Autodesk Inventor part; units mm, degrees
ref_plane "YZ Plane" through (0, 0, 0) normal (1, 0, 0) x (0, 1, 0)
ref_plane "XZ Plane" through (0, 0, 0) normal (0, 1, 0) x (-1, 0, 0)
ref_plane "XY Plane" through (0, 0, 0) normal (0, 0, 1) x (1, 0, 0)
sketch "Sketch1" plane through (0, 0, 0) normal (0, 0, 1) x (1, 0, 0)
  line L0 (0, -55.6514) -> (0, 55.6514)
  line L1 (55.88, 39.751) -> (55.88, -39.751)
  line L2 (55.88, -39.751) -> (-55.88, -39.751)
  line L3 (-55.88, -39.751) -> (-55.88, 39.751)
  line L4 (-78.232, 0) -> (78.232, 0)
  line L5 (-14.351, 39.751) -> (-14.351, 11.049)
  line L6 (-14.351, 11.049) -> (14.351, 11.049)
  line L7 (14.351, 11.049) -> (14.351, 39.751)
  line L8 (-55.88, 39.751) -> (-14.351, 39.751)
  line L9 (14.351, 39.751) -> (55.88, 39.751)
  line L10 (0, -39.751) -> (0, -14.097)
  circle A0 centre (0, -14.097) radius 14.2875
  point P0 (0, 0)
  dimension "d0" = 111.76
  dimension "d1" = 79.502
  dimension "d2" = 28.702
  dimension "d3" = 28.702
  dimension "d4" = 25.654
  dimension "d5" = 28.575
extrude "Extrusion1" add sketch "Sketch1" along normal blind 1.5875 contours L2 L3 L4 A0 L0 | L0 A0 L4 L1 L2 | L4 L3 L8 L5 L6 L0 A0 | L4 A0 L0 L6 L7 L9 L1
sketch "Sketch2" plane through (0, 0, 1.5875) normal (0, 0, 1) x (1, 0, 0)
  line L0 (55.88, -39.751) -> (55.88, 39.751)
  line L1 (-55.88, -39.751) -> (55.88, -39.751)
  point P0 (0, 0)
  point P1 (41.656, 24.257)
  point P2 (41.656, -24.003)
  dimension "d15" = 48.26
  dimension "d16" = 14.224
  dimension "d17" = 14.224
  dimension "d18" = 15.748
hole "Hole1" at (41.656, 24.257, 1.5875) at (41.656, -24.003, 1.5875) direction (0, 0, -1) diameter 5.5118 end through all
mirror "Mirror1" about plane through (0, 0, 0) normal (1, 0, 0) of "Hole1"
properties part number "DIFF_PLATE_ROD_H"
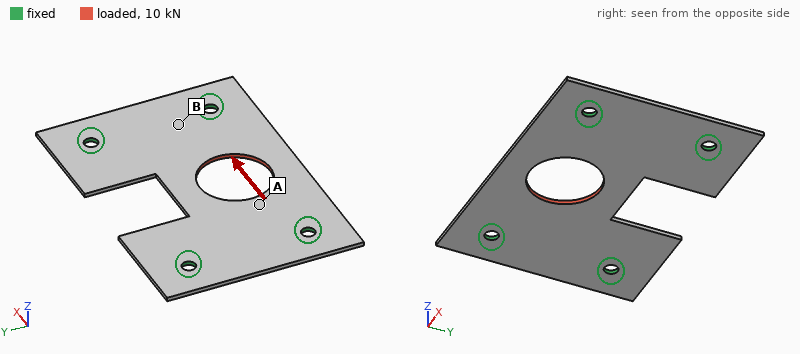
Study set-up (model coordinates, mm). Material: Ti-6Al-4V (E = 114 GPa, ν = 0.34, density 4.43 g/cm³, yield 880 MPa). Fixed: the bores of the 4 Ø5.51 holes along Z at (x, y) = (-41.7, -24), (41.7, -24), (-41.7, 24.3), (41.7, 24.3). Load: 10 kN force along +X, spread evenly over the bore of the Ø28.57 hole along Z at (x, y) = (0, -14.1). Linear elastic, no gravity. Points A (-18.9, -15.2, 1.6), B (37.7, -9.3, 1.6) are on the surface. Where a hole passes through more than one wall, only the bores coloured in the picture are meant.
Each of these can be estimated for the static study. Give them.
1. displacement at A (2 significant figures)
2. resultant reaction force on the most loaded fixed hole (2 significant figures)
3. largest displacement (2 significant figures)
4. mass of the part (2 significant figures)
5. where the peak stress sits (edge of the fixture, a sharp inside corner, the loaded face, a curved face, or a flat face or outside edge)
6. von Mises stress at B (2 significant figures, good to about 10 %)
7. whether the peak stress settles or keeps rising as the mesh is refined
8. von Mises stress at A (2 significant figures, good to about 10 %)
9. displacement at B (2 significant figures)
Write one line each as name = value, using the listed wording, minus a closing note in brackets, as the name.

displacement at A = 20 µm
resultant reaction force on the most loaded fixed hole = 3.7 kN
largest displacement = 30 µm
mass of the part = 52 g
where the peak stress sits = edge of the fixture
von Mises stress at B = 36 MPa
whether the peak stress settles or keeps rising as the mesh is refined = keeps rising
von Mises stress at A = 73 MPa
displacement at B = 13 µm
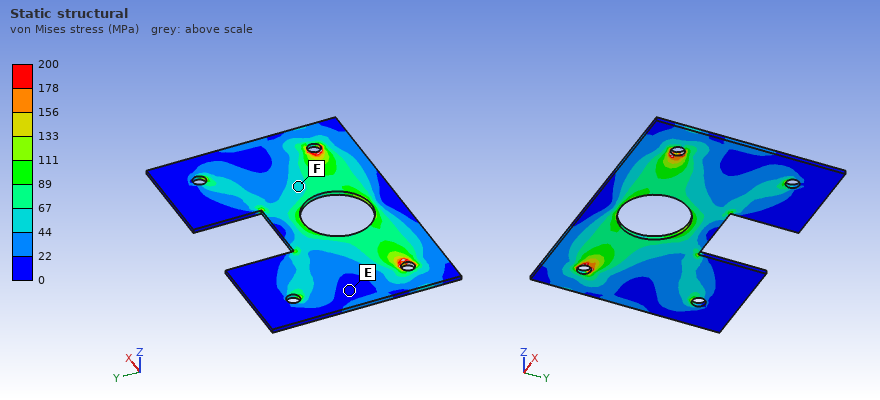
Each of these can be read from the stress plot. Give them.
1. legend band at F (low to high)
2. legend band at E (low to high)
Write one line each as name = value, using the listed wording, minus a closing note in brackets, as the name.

legend band at F = 44 to 67 MPa
legend band at E = 0 to 22 MPa
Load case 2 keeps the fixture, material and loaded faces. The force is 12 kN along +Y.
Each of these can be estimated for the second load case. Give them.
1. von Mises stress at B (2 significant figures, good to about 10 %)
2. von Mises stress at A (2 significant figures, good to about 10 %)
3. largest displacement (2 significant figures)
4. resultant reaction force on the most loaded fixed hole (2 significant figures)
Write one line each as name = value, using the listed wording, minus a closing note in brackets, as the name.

von Mises stress at B = 85 MPa
von Mises stress at A = 180 MPa
largest displacement = 98 µm
resultant reaction force on the most loaded fixed hole = 4.0 kN
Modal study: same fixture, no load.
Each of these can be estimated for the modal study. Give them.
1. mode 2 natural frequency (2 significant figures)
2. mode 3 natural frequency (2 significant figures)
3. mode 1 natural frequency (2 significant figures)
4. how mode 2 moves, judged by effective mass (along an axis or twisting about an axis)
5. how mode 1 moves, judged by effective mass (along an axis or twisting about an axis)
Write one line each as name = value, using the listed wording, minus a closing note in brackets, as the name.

mode 2 natural frequency = 1700 Hz
mode 3 natural frequency = 2400 Hz
mode 1 natural frequency = 1300 Hz
how mode 2 moves, judged by effective mass = twisting about X
how mode 1 moves, judged by effective mass = along Z
